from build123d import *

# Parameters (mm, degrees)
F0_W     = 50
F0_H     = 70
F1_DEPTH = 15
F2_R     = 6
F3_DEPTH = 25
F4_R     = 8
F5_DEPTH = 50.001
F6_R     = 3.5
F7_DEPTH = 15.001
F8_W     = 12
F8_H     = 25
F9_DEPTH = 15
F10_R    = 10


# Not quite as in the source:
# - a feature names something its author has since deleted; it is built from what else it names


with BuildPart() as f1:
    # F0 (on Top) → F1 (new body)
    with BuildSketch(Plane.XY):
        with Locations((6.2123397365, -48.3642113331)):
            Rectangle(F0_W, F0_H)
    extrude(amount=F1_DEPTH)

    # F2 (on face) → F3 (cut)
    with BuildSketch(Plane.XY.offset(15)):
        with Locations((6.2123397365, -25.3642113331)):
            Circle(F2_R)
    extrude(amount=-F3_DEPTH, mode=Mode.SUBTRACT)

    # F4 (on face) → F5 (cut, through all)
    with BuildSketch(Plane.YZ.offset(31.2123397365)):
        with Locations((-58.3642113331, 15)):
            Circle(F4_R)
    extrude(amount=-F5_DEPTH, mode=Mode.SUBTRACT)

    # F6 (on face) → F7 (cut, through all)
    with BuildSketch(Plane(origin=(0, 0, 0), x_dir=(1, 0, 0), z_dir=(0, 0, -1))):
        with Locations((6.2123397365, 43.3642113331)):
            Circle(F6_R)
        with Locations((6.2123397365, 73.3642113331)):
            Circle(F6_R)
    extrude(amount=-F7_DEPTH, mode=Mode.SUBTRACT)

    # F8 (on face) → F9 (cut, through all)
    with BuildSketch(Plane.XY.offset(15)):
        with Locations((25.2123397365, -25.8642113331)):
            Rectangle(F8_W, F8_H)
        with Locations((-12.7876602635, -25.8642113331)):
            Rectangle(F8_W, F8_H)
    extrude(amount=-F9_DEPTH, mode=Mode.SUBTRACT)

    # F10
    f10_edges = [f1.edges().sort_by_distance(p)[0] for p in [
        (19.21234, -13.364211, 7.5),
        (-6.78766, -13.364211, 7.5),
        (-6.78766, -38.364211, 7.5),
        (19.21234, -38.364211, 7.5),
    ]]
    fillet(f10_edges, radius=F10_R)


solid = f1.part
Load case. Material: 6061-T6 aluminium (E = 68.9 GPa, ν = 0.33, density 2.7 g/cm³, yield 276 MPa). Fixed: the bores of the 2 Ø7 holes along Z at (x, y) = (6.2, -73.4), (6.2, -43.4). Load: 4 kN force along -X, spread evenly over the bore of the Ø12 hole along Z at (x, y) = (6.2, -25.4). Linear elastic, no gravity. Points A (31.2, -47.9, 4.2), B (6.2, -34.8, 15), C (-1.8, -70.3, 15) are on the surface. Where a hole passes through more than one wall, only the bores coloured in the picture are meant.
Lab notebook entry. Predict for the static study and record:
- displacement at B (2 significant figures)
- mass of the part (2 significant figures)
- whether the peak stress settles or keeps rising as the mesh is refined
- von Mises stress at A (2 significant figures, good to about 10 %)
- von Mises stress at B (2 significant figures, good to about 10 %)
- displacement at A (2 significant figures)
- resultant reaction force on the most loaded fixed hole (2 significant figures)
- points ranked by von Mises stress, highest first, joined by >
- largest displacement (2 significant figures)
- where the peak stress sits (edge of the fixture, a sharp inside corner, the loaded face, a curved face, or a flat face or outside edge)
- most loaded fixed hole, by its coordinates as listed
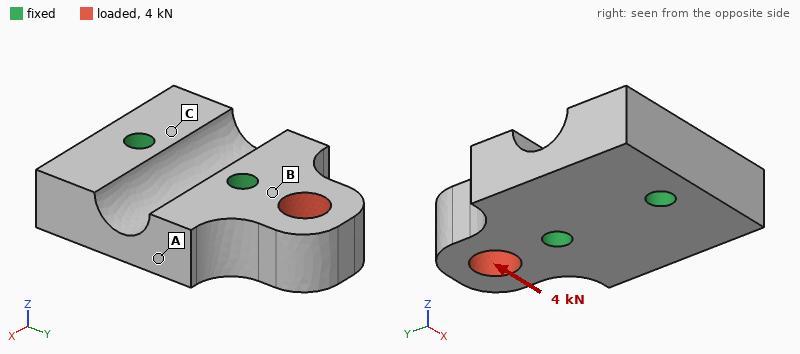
5.0 µm
96 g
keeps rising
9.9 MPa
28 MPa
5.8 µm
5.5 kN
B > A > C
29 µm
edge of the fixture
(6.2, -43.4)
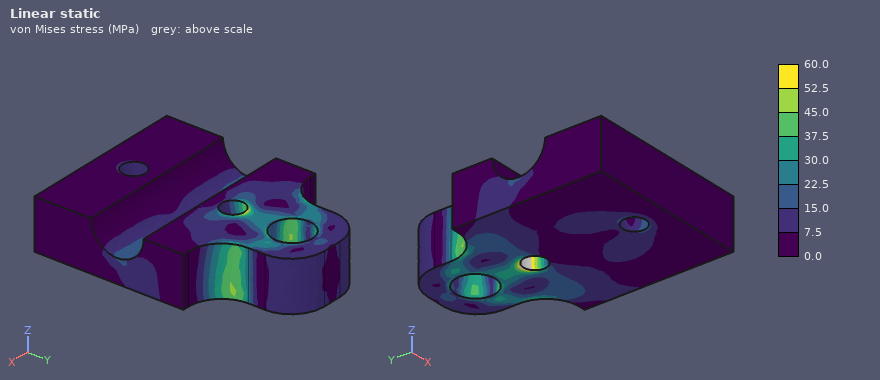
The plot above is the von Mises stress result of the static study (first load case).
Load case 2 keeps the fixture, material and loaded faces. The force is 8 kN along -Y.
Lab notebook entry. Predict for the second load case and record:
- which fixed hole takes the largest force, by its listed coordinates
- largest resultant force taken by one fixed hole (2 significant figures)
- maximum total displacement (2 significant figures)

(6.2, -43.4)
6.8 kN
14 µm
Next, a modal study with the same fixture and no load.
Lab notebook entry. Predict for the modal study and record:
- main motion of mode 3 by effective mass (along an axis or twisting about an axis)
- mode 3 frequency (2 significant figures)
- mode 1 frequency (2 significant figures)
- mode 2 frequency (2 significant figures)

twisting about Y
16 kHz
13 kHz
15 kHz
